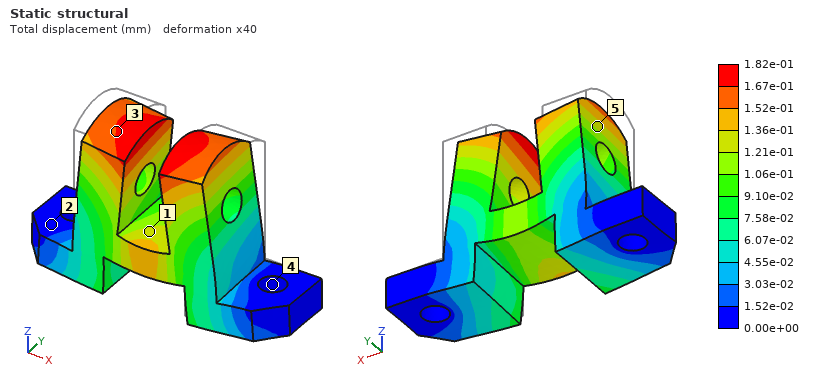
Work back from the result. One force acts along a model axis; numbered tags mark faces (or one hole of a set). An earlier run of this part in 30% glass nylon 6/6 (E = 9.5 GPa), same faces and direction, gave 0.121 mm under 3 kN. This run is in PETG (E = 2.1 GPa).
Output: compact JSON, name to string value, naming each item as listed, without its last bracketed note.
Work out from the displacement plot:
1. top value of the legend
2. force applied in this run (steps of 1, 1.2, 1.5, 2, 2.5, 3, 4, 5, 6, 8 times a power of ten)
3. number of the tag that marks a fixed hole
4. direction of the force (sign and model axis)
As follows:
{"top value of the legend": "1.82e-01 mm", "force applied in this run": "1 kN", "number of the tag that marks a fixed hole": "4", "direction of the force": "-Z"}
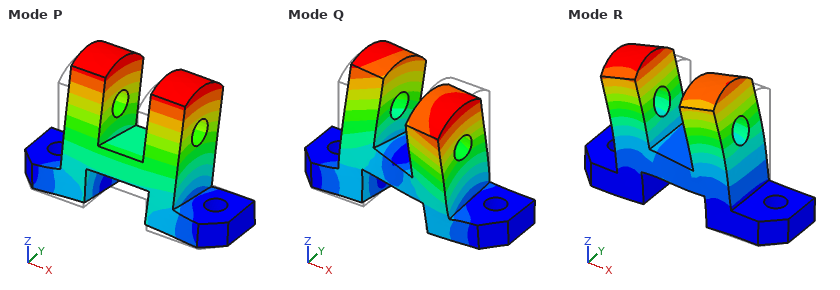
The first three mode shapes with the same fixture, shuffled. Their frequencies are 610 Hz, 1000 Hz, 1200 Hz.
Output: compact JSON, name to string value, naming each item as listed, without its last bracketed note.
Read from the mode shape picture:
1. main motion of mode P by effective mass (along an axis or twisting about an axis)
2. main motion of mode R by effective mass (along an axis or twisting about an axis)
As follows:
{"main motion of mode P by effective mass": "along Y", "main motion of mode R by effective mass": "along X"}
